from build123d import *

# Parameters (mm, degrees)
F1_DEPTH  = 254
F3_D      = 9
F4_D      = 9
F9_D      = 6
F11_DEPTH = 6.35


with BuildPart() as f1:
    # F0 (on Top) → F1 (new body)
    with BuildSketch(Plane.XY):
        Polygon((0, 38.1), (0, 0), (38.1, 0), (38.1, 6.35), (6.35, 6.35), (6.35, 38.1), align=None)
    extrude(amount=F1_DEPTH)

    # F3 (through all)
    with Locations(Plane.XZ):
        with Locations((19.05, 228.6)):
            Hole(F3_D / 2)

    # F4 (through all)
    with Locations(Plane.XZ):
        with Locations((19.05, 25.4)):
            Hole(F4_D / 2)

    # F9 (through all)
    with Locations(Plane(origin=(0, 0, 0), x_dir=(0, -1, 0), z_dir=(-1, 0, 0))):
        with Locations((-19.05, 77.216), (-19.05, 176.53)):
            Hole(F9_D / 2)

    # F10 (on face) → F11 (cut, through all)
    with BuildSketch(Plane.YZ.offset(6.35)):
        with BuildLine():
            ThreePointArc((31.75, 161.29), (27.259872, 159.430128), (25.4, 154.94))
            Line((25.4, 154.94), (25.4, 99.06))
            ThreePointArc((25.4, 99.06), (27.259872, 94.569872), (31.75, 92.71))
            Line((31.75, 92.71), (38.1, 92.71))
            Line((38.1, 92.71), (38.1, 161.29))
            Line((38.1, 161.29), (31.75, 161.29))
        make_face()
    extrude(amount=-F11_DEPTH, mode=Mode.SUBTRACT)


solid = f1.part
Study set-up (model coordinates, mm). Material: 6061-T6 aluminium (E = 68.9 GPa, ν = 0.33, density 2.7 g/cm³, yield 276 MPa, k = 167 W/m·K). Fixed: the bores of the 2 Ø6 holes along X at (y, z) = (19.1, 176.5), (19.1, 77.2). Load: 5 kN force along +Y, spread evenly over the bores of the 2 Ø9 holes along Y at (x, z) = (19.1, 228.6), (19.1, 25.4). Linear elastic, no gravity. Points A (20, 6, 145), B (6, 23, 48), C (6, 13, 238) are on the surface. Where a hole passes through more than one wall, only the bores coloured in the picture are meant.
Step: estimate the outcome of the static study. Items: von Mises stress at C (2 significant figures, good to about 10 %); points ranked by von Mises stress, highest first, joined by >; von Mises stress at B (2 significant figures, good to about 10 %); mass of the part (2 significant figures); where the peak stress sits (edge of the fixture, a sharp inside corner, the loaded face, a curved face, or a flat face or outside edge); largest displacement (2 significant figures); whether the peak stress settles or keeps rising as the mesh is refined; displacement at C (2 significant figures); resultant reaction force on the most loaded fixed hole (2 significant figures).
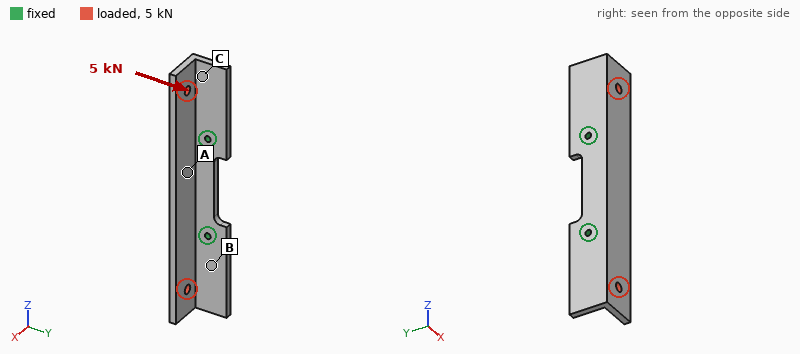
55 MPa
B > C > A
84 MPa
290 g
edge of the fixture
0.96 mm
keeps rising
0.28 mm
4.9 kN
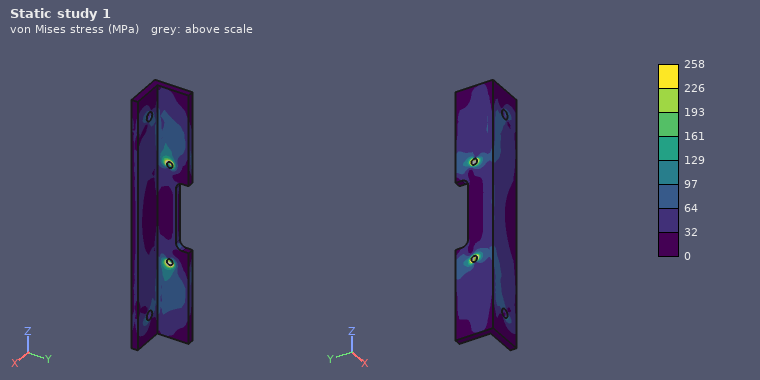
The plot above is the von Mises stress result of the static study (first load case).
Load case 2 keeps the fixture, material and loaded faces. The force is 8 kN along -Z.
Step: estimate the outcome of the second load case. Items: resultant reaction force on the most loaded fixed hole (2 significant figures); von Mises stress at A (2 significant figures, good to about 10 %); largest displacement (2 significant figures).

4.3 kN
19 MPa
0.13 mm
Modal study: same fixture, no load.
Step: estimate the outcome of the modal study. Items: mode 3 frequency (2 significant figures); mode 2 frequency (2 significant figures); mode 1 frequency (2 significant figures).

1900 Hz
1500 Hz
1500 Hz
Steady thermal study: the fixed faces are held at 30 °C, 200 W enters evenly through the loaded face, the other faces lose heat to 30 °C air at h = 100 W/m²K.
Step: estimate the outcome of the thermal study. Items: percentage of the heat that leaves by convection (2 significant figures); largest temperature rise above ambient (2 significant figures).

54 %
79 K
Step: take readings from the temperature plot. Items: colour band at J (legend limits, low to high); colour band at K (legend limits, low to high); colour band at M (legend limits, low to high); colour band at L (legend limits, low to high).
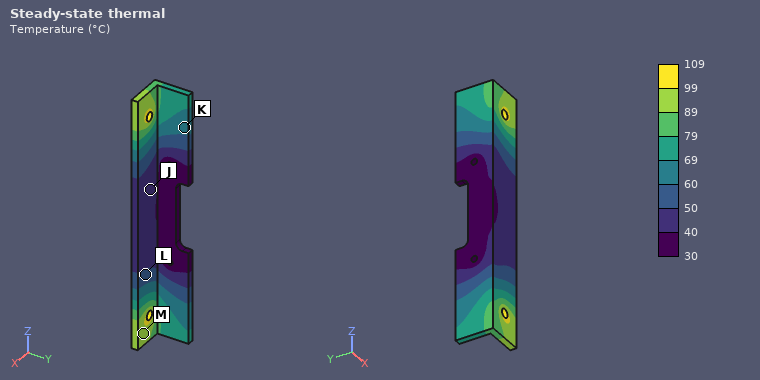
40 to 50 °C
60 to 69 °C
89 to 99 °C
50 to 60 °C
